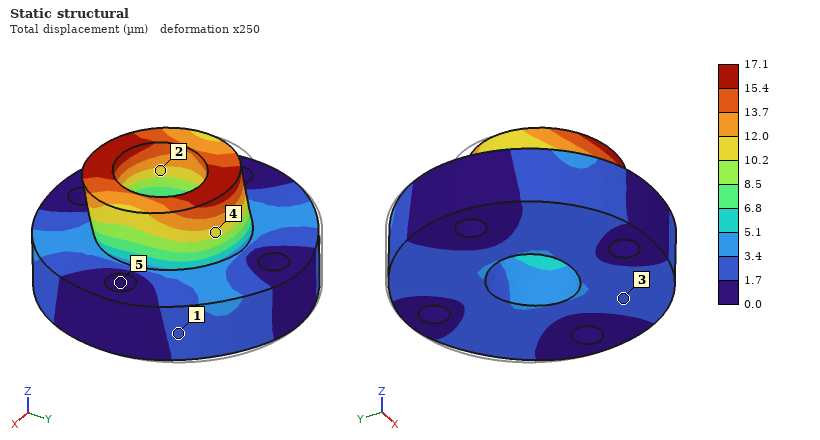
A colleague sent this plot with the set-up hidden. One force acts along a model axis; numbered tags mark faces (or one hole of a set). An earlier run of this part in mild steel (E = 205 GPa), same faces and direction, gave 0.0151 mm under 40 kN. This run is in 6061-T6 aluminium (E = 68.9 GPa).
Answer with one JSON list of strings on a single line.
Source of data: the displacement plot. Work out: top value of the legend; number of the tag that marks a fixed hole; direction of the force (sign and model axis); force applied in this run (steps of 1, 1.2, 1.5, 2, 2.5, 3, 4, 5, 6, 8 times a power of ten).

["17.1 µm", "5", "-Y", "15 kN"]
